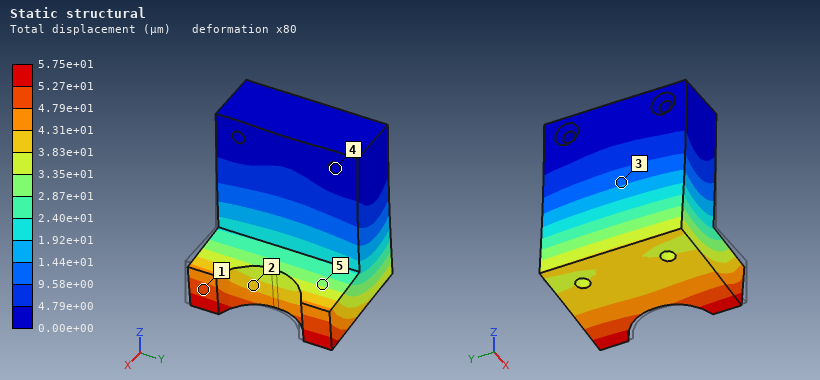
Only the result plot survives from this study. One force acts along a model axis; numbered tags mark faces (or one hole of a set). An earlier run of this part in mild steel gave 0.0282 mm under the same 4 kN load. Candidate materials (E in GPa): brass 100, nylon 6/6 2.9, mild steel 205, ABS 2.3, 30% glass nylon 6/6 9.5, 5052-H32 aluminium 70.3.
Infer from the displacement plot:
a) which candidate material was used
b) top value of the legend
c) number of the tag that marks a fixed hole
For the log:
brass
5.75e+01 µm
4
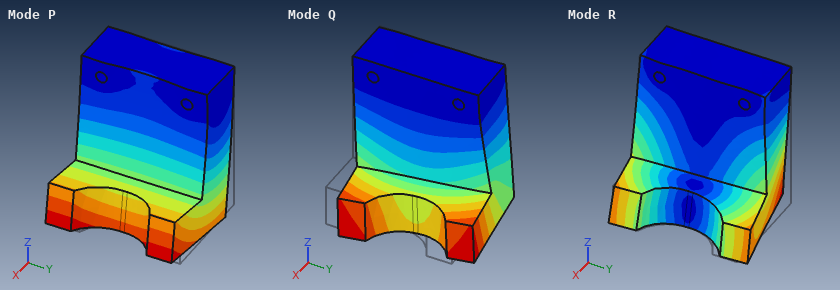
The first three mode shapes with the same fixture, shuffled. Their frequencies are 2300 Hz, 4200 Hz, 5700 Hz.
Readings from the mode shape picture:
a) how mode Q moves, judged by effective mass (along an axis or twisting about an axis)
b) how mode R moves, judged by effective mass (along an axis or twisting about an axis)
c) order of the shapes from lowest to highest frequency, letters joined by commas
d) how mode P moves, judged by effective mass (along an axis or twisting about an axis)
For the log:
along Y
along Y
P, Q, R
along X
